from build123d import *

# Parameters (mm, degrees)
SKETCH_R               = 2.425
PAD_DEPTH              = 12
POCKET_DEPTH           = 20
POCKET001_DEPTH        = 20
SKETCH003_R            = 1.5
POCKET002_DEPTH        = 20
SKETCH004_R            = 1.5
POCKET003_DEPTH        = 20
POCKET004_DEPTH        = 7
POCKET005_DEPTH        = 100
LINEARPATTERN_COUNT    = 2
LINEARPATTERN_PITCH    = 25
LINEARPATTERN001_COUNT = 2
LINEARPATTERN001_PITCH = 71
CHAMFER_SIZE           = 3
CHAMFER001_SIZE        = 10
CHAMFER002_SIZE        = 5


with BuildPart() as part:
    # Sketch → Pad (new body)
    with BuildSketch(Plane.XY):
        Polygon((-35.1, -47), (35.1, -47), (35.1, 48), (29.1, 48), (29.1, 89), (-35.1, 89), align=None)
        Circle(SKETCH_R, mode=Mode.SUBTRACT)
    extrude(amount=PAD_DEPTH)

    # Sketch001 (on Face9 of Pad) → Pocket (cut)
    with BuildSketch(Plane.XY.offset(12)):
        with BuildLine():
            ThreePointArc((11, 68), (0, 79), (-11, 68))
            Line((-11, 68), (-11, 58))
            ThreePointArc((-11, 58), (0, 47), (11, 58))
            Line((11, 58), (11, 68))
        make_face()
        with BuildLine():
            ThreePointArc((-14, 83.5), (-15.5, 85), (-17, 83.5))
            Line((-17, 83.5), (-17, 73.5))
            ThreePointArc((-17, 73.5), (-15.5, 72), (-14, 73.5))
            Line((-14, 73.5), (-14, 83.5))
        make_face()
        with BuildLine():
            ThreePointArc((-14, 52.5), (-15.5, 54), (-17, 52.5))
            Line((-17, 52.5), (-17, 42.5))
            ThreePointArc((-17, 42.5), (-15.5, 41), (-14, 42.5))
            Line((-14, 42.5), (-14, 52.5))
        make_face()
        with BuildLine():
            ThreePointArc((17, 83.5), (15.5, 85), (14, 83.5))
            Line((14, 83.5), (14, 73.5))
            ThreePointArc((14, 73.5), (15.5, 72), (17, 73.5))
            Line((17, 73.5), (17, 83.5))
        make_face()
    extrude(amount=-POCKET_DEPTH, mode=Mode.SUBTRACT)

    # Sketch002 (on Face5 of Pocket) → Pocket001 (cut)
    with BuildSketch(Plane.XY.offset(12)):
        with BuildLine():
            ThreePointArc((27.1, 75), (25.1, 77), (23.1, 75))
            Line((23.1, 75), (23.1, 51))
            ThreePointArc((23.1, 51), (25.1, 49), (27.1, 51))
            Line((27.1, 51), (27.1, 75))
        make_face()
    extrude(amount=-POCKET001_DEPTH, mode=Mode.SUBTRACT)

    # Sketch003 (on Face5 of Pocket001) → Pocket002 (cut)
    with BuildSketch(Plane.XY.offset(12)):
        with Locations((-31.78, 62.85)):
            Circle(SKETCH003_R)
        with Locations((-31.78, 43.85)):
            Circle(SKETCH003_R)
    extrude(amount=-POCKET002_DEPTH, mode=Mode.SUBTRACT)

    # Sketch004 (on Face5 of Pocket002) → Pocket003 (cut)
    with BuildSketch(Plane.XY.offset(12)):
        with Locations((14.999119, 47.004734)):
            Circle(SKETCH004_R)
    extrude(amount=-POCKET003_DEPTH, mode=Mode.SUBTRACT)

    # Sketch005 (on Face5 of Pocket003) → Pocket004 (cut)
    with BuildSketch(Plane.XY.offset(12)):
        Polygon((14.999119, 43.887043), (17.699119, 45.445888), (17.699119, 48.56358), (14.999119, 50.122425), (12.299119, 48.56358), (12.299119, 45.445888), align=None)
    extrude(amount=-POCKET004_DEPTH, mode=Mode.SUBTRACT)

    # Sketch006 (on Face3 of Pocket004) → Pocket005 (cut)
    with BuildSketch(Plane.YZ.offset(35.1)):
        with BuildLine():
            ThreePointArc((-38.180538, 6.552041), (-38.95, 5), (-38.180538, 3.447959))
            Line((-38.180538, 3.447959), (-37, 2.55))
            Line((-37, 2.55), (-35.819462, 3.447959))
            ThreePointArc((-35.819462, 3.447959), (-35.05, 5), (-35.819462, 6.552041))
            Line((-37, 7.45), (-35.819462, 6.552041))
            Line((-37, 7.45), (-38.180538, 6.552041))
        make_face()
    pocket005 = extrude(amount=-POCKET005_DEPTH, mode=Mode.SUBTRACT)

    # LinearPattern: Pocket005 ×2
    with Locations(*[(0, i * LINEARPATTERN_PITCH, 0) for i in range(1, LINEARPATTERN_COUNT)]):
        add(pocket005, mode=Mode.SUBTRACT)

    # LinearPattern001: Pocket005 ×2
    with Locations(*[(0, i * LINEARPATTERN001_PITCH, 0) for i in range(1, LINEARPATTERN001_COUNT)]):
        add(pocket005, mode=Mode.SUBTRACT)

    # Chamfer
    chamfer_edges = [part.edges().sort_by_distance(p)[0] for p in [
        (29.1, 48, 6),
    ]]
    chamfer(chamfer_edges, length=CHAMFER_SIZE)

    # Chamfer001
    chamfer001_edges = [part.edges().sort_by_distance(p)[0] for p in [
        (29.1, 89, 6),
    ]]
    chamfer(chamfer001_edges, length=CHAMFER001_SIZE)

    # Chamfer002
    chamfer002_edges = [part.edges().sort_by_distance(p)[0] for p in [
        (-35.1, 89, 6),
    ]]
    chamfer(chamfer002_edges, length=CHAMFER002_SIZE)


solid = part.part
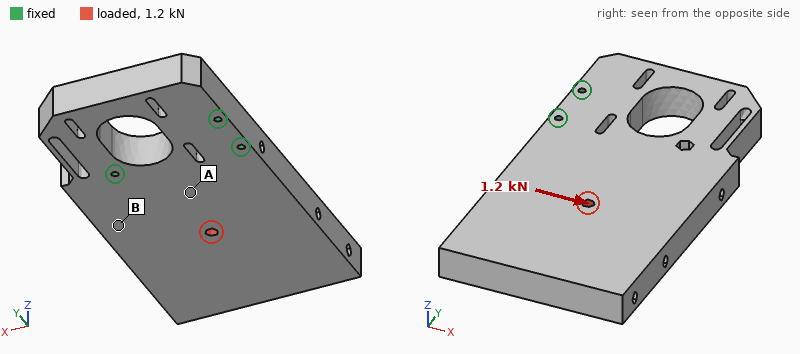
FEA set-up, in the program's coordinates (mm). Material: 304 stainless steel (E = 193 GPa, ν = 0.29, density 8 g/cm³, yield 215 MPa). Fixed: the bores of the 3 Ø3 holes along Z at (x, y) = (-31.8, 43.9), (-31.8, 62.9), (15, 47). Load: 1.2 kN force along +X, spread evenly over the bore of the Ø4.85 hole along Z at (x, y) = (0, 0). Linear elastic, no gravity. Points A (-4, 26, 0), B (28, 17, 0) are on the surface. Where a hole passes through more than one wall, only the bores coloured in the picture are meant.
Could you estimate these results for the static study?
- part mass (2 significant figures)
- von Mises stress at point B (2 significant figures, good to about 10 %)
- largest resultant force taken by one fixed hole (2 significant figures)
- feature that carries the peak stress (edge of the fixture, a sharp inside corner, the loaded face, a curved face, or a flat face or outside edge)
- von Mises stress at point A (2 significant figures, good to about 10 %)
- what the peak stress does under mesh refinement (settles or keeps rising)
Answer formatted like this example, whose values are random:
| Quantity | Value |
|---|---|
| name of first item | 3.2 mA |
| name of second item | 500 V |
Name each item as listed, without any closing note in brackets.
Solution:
| Quantity | Value |
|---|---|
| part mass | 780 g |
| von Mises stress at point B | 2.1 MPa |
| largest resultant force taken by one fixed hole | 1.2 kN |
| feature that carries the peak stress | edge of the fixture |
| von Mises stress at point A | 4.7 MPa |
| what the peak stress does under mesh refinement | keeps rising |
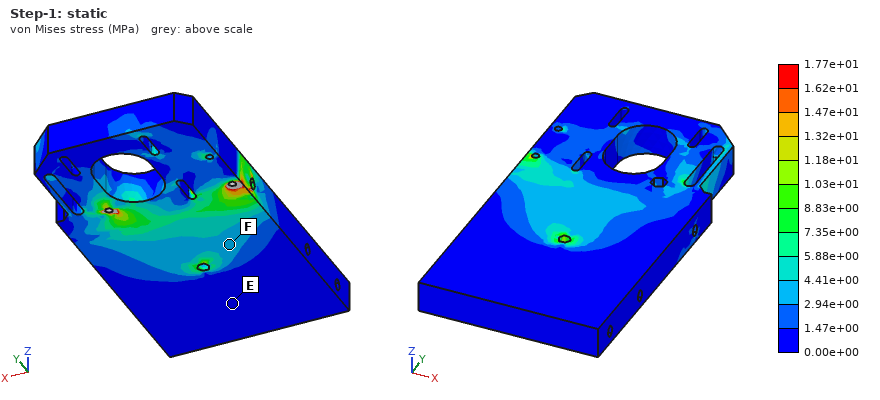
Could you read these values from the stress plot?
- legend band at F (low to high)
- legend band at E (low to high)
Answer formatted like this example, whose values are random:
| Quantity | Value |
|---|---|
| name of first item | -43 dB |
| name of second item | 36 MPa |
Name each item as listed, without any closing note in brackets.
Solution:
| Quantity | Value |
|---|---|
| legend band at F | 2.94e+00 to 4.41e+00 MPa |
| legend band at E | 0.00e+00 to 1.47e+00 MPa |
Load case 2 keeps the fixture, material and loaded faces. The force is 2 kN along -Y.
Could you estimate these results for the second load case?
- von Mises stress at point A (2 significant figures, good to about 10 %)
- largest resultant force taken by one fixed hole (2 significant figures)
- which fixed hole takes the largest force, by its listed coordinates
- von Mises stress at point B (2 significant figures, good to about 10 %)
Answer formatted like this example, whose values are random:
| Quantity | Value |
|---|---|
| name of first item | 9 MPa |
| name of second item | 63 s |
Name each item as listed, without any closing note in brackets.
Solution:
| Quantity | Value |
|---|---|
| von Mises stress at point A | 3.2 MPa |
| largest resultant force taken by one fixed hole | 1.2 kN |
| which fixed hole takes the largest force, by its listed coordinates | (15, 47) |
| von Mises stress at point B | 2.3 MPa |
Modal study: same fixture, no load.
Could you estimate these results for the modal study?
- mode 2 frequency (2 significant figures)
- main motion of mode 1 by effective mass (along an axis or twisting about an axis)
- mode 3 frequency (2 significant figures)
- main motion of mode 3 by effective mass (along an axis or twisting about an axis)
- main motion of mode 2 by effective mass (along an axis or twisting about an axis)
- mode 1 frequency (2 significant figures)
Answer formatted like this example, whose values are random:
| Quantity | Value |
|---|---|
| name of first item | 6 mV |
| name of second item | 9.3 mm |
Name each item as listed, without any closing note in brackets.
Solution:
| Quantity | Value |
|---|---|
| mode 2 frequency | 2800 Hz |
| main motion of mode 1 by effective mass | along Z |
| mode 3 frequency | 3400 Hz |
| main motion of mode 3 by effective mass | along X |
| main motion of mode 2 by effective mass | twisting about Y |
| mode 1 frequency | 790 Hz |
